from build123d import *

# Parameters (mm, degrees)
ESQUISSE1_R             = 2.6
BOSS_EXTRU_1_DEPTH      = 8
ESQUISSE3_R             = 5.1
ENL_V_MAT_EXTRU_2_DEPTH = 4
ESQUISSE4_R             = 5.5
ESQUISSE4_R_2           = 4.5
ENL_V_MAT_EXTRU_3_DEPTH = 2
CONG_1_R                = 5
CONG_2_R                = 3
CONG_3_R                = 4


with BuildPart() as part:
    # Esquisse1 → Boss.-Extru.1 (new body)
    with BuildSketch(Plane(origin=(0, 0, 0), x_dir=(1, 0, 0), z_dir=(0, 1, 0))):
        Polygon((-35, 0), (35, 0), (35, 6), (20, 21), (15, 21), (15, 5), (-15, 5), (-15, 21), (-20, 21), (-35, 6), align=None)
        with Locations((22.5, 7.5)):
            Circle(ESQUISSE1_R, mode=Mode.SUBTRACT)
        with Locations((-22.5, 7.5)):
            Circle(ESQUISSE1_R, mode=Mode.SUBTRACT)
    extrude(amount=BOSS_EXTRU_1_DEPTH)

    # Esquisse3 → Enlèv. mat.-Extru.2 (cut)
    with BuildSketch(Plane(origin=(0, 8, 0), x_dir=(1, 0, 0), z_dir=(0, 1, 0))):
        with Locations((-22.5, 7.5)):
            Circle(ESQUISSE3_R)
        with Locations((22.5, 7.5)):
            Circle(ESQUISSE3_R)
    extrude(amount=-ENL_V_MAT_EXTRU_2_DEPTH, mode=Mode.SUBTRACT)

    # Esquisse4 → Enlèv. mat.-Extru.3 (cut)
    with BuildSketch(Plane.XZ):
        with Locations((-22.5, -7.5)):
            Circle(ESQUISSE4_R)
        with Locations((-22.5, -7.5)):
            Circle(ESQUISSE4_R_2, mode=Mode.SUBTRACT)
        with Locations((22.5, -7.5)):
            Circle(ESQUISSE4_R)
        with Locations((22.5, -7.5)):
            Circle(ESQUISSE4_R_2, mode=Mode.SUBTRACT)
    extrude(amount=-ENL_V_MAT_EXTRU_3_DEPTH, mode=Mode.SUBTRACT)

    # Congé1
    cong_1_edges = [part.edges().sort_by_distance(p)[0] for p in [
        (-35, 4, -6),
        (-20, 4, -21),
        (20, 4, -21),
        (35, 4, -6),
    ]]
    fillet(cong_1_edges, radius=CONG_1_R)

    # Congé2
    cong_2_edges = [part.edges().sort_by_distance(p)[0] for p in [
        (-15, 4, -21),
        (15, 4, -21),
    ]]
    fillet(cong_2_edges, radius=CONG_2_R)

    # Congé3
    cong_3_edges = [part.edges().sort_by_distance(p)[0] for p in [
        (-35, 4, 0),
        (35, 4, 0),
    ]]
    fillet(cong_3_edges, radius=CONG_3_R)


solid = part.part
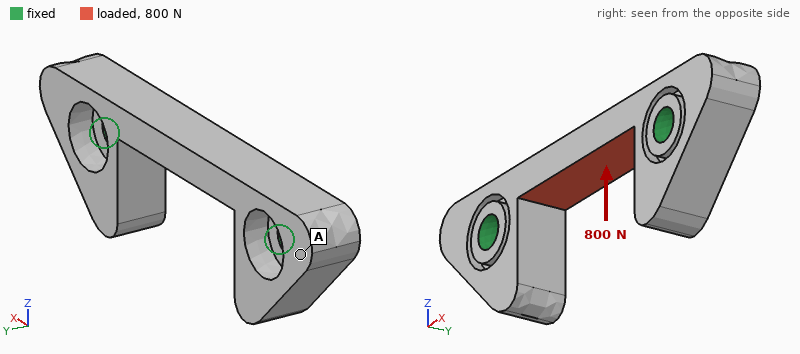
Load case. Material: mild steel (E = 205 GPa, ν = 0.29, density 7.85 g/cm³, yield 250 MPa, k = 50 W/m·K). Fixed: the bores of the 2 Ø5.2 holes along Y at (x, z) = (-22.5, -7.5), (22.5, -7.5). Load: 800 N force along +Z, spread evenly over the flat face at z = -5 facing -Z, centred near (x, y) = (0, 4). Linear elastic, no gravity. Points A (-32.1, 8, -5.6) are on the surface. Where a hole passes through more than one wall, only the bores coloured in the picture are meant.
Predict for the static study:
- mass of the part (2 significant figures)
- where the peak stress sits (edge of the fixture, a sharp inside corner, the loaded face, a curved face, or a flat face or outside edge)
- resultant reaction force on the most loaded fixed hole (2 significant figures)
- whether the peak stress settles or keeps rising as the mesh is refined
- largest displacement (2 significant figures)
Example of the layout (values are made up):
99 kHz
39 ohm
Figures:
40 g
edge of the fixture
480 N
keeps rising
11 µm
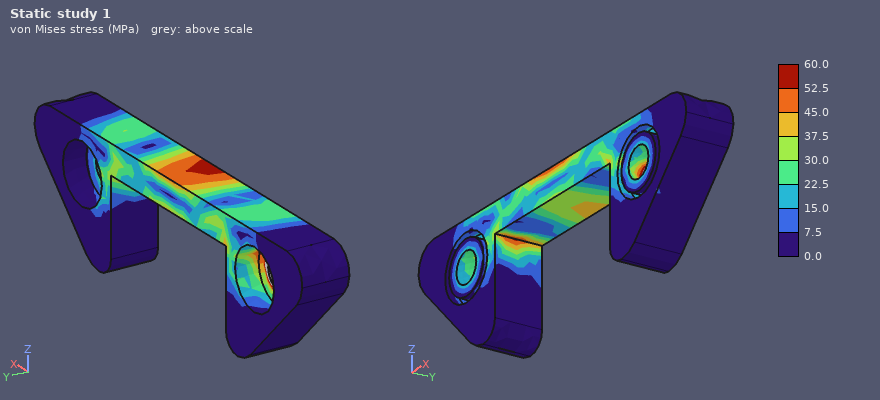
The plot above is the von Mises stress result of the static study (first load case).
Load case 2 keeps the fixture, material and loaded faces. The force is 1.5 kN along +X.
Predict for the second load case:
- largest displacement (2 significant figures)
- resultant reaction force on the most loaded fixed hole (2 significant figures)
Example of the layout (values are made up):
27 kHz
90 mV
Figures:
3.2 µm
760 N
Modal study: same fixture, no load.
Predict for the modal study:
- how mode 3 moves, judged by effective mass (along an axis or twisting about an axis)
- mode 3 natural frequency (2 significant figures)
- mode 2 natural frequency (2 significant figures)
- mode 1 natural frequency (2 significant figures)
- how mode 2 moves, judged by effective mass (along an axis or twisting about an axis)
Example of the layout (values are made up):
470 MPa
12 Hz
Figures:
twisting about X
17 kHz
16 kHz
13 kHz
along Z
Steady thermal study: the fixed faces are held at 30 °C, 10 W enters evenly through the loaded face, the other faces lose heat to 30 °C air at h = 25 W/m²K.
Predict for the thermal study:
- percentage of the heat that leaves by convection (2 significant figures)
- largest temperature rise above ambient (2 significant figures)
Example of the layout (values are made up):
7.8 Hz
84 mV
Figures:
6.7 %
36 K
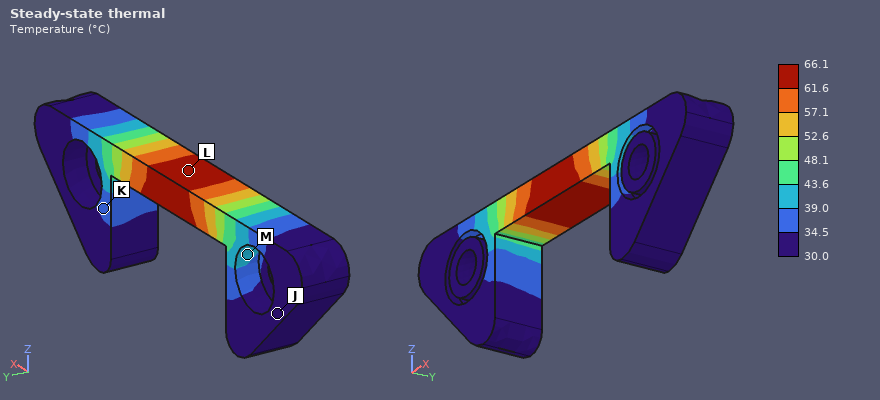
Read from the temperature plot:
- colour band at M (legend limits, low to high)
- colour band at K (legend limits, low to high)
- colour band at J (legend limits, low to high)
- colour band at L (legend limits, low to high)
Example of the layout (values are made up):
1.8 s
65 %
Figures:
39.0 to 43.6 °C
34.5 to 39.0 °C
30.0 to 34.5 °C
61.6 to 66.1 °C
